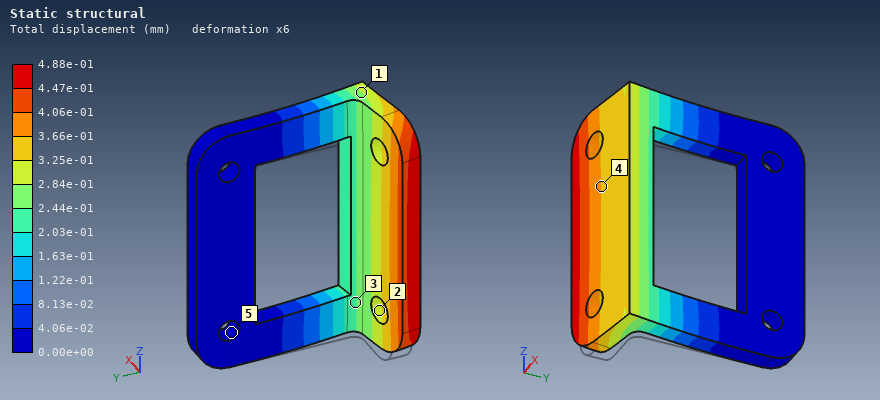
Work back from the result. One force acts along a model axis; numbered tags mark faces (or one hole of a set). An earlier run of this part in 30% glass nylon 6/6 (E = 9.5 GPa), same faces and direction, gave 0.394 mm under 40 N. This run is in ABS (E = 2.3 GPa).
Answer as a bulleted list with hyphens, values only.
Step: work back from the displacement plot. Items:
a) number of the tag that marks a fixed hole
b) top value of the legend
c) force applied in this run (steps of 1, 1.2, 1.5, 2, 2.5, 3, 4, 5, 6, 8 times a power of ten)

- 5
- 4.88e-01 mm
- 12 N
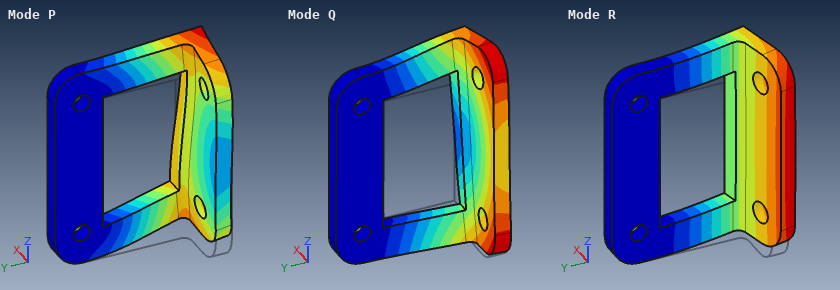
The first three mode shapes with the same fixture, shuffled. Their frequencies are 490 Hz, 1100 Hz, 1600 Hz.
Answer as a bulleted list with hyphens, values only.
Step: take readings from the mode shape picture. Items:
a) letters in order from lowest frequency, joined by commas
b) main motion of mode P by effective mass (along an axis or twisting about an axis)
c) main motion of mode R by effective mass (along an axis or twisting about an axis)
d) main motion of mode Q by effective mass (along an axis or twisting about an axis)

- R, Q, P
- along Z
- along X
- along Z
